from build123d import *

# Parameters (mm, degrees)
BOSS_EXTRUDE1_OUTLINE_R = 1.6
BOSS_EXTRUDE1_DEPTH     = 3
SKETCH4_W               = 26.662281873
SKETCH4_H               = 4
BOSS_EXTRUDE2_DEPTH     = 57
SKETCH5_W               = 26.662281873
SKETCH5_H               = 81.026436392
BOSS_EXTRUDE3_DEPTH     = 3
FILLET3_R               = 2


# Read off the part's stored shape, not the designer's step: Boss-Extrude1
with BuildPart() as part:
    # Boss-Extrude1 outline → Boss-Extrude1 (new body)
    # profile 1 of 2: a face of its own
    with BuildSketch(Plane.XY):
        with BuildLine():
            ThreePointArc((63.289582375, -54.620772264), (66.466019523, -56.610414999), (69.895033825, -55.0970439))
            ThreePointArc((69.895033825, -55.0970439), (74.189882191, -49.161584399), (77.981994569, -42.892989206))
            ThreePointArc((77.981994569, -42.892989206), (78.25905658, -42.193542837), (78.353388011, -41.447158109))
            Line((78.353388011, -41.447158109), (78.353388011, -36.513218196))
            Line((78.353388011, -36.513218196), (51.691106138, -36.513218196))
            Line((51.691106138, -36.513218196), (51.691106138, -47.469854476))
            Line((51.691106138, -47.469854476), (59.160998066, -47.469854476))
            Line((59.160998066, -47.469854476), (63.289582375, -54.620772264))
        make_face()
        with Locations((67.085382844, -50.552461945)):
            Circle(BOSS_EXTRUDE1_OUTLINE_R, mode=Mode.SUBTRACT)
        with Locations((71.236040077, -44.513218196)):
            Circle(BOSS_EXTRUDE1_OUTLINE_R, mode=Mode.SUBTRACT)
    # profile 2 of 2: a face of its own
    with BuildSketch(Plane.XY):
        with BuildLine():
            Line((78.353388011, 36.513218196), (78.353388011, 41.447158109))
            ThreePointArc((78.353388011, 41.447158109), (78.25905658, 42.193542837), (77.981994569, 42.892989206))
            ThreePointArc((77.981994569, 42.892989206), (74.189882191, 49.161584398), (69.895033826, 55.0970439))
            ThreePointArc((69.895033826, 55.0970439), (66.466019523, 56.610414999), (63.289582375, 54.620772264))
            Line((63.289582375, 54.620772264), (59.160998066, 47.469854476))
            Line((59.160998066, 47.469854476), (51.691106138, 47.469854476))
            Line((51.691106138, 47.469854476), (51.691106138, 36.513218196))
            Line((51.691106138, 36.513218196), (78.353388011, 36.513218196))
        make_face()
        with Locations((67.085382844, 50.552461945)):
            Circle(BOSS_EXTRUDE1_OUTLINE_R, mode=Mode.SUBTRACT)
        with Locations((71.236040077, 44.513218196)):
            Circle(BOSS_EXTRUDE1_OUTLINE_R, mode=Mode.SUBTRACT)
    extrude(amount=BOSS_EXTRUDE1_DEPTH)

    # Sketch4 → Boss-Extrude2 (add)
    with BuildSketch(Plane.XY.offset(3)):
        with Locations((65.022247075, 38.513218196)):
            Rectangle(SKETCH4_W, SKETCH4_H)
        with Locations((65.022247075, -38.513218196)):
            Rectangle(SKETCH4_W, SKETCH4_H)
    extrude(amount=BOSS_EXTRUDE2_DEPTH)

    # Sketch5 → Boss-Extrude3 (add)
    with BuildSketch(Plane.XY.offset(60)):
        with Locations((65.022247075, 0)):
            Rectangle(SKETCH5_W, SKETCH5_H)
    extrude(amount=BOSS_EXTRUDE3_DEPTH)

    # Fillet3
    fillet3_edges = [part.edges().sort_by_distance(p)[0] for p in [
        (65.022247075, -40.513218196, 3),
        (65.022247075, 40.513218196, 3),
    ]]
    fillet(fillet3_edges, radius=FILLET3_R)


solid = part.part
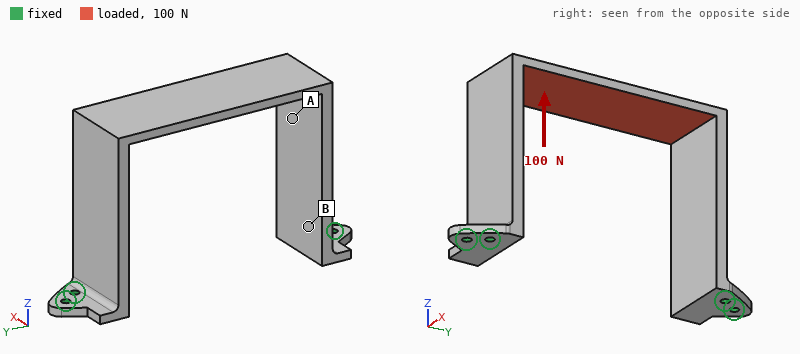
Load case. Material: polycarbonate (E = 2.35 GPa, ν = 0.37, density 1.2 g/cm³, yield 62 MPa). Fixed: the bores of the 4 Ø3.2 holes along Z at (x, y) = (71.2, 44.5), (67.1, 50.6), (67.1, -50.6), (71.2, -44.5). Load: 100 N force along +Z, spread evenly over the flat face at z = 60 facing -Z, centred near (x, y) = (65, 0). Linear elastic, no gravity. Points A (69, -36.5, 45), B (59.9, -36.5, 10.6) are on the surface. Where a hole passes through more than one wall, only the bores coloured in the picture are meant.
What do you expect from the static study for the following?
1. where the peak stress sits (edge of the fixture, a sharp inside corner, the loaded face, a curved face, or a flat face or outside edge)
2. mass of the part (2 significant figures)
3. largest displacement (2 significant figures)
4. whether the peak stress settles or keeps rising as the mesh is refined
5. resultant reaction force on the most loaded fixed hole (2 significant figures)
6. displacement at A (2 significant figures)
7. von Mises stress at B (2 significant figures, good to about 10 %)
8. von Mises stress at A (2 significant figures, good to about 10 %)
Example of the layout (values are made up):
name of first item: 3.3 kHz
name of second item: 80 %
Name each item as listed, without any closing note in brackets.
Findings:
where the peak stress sits: edge of the fixture
mass of the part: 25 g
largest displacement: 1.4 mm
whether the peak stress settles or keeps rising as the mesh is refined: keeps rising
resultant reaction force on the most loaded fixed hole: 31 N
displacement at A: 0.33 mm
von Mises stress at B: 1.6 MPa
von Mises stress at A: 5.2 MPa
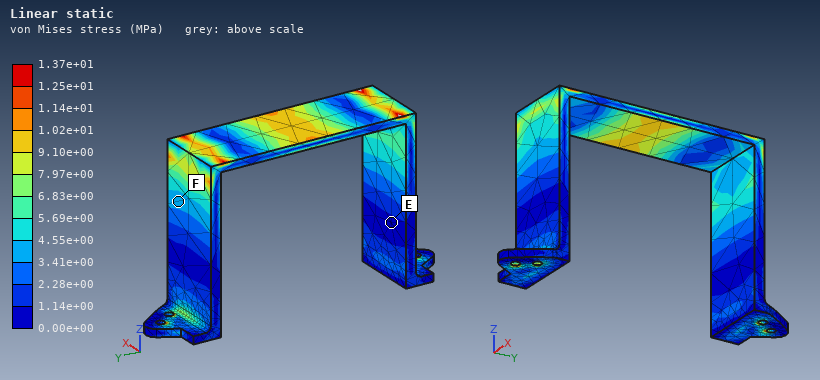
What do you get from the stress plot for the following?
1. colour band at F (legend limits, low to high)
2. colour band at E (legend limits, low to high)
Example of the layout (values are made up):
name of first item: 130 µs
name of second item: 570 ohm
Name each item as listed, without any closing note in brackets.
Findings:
colour band at F: 3.41e+00 to 4.55e+00 MPa
colour band at E: 0.00e+00 to 1.14e+00 MPa
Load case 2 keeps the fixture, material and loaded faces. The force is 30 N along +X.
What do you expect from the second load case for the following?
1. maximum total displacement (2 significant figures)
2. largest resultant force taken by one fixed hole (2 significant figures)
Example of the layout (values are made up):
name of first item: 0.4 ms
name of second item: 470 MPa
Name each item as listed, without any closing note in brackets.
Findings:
maximum total displacement: 1.4 mm
largest resultant force taken by one fixed hole: 44 N
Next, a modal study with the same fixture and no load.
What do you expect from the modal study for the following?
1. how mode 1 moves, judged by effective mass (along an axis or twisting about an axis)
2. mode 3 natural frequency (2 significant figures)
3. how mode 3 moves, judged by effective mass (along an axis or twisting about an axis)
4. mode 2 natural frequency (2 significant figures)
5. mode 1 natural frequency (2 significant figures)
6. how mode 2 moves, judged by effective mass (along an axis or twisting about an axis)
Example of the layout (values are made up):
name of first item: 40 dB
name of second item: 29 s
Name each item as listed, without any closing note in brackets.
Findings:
how mode 1 moves, judged by effective mass: along Y
mode 3 natural frequency: 320 Hz
how mode 3 moves, judged by effective mass: twisting about Z
mode 2 natural frequency: 210 Hz
mode 1 natural frequency: 170 Hz
how mode 2 moves, judged by effective mass: along X
